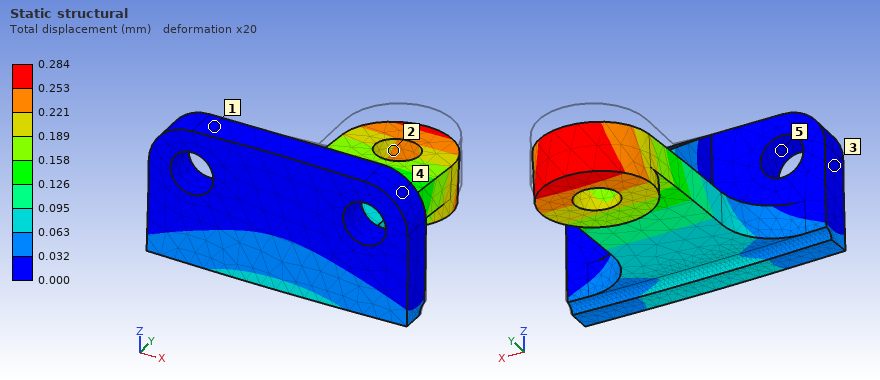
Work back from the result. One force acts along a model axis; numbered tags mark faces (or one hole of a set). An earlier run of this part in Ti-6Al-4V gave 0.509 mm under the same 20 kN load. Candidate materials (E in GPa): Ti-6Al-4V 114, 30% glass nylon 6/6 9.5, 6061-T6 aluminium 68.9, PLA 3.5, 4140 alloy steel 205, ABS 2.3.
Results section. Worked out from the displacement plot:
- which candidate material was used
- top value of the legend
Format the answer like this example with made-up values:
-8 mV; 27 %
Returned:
4140 alloy steel; 0.284 mm
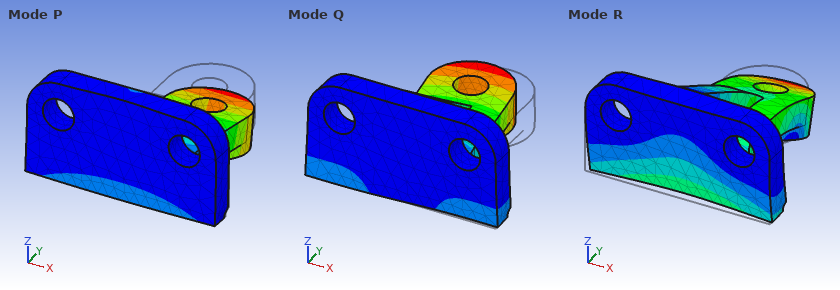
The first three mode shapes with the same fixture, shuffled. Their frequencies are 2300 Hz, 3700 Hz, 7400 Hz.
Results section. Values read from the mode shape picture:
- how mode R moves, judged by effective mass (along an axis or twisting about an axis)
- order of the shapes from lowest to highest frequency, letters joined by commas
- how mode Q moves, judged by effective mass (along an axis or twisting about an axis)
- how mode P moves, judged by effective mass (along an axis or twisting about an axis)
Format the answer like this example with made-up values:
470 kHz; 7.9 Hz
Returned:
along Y; P, Q, R; along X; along Z
